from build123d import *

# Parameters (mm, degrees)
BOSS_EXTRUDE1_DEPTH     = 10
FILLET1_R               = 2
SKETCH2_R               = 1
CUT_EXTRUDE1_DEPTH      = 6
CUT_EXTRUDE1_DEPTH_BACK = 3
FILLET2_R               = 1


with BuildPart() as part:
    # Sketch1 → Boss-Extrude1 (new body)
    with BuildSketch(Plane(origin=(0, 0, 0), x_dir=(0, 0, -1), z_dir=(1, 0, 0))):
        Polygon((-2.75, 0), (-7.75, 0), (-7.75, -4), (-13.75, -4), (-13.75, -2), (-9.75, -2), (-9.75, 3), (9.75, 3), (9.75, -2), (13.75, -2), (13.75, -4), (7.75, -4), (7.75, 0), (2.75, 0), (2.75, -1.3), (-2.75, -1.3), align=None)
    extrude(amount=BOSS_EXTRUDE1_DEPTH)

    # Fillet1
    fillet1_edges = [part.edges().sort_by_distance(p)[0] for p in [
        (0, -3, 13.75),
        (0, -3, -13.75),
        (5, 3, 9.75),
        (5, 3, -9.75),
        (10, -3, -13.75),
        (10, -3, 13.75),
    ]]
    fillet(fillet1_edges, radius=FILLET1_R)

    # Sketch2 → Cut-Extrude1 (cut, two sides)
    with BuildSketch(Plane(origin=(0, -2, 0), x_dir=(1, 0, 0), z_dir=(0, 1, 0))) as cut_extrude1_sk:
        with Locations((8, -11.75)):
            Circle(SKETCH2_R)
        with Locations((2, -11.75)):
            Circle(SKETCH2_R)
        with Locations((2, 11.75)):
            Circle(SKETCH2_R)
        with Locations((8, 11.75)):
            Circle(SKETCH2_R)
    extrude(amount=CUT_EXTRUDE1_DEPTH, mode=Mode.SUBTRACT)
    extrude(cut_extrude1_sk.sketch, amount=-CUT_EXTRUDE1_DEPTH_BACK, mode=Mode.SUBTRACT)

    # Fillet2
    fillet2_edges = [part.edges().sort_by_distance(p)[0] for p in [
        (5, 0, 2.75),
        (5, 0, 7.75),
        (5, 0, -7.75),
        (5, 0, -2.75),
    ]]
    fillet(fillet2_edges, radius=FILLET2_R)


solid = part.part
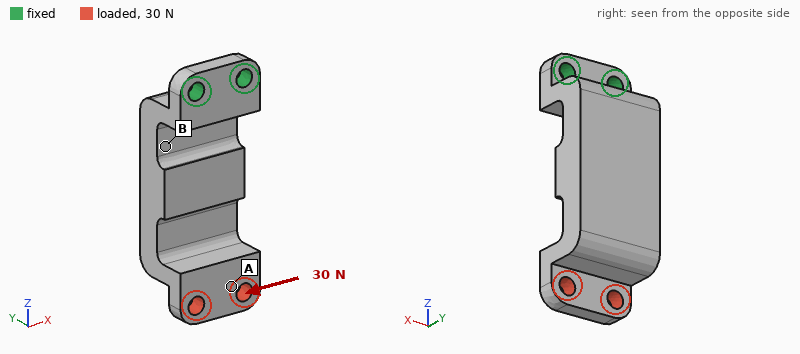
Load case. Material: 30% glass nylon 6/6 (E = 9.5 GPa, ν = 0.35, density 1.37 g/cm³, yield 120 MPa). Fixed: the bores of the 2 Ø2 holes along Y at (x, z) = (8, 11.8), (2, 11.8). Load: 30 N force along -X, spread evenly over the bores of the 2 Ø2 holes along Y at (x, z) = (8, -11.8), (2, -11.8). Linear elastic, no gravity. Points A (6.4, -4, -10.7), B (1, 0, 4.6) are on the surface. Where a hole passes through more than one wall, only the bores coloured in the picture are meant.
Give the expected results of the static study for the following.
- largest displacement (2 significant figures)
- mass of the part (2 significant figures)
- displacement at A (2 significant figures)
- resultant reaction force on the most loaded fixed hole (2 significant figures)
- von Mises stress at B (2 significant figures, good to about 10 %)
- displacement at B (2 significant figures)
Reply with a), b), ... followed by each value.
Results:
a) 0.36 mm
b) 1.3 g
c) 0.31 mm
d) 100 N
e) 21 MPa
f) 0.074 mm
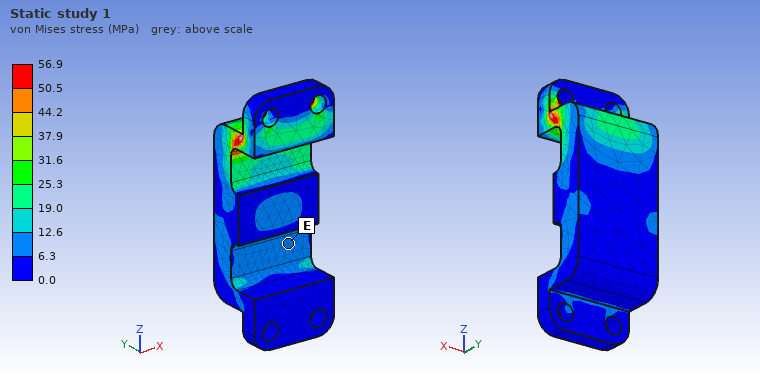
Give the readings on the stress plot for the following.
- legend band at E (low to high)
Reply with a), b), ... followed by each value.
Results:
a) 6.3 to 12.6 MPa
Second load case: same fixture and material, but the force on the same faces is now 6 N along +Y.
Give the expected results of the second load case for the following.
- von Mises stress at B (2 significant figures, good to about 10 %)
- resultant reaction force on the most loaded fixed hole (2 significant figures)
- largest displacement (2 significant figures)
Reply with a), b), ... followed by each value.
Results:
a) 6.1 MPa
b) 3.3 N
c) 0.31 mm
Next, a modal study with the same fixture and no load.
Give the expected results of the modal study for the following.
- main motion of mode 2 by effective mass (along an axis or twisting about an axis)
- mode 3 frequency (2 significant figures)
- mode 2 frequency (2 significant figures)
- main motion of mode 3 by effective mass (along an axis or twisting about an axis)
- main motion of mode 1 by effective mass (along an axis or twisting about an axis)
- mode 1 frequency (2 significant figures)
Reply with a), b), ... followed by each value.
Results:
a) along X
b) 7000 Hz
c) 2700 Hz
d) along Z
e) along Y
f) 1200 Hz
